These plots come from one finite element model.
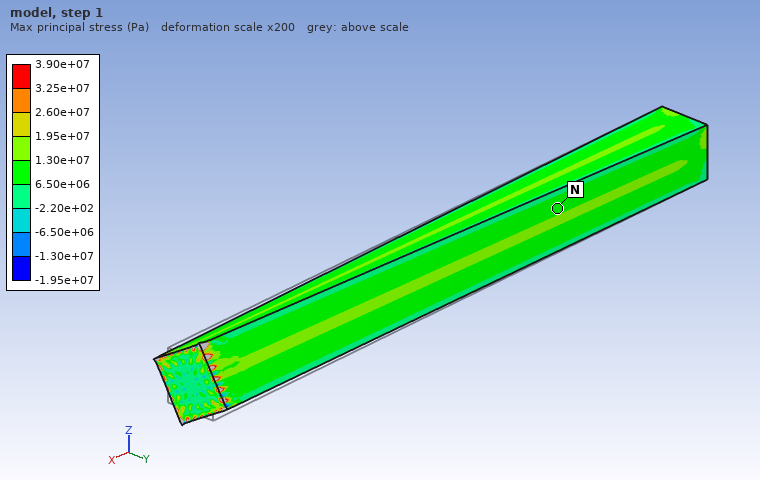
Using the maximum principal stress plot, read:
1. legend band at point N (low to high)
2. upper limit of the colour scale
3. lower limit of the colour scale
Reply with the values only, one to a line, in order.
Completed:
6.50e+06 to 1.30e+07 Pa
3.90e+07 Pa
-1.95e+07 Pa
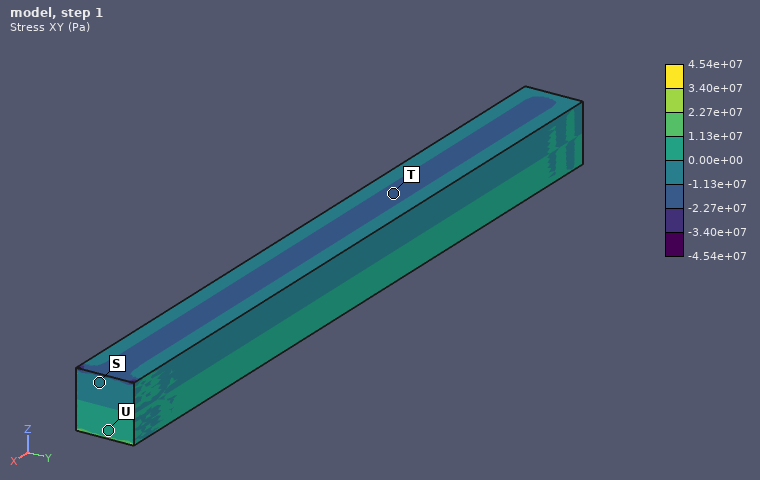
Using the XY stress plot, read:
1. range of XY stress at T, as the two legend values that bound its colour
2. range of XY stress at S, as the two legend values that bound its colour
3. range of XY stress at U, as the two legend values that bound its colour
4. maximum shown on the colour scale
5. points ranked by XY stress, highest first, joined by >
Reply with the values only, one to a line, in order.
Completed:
-2.27e+07 to -1.13e+07 Pa
-1.13e+07 to 0.00e+00 Pa
0.00e+00 to 1.13e+07 Pa
4.54e+07 Pa
U > S > T
